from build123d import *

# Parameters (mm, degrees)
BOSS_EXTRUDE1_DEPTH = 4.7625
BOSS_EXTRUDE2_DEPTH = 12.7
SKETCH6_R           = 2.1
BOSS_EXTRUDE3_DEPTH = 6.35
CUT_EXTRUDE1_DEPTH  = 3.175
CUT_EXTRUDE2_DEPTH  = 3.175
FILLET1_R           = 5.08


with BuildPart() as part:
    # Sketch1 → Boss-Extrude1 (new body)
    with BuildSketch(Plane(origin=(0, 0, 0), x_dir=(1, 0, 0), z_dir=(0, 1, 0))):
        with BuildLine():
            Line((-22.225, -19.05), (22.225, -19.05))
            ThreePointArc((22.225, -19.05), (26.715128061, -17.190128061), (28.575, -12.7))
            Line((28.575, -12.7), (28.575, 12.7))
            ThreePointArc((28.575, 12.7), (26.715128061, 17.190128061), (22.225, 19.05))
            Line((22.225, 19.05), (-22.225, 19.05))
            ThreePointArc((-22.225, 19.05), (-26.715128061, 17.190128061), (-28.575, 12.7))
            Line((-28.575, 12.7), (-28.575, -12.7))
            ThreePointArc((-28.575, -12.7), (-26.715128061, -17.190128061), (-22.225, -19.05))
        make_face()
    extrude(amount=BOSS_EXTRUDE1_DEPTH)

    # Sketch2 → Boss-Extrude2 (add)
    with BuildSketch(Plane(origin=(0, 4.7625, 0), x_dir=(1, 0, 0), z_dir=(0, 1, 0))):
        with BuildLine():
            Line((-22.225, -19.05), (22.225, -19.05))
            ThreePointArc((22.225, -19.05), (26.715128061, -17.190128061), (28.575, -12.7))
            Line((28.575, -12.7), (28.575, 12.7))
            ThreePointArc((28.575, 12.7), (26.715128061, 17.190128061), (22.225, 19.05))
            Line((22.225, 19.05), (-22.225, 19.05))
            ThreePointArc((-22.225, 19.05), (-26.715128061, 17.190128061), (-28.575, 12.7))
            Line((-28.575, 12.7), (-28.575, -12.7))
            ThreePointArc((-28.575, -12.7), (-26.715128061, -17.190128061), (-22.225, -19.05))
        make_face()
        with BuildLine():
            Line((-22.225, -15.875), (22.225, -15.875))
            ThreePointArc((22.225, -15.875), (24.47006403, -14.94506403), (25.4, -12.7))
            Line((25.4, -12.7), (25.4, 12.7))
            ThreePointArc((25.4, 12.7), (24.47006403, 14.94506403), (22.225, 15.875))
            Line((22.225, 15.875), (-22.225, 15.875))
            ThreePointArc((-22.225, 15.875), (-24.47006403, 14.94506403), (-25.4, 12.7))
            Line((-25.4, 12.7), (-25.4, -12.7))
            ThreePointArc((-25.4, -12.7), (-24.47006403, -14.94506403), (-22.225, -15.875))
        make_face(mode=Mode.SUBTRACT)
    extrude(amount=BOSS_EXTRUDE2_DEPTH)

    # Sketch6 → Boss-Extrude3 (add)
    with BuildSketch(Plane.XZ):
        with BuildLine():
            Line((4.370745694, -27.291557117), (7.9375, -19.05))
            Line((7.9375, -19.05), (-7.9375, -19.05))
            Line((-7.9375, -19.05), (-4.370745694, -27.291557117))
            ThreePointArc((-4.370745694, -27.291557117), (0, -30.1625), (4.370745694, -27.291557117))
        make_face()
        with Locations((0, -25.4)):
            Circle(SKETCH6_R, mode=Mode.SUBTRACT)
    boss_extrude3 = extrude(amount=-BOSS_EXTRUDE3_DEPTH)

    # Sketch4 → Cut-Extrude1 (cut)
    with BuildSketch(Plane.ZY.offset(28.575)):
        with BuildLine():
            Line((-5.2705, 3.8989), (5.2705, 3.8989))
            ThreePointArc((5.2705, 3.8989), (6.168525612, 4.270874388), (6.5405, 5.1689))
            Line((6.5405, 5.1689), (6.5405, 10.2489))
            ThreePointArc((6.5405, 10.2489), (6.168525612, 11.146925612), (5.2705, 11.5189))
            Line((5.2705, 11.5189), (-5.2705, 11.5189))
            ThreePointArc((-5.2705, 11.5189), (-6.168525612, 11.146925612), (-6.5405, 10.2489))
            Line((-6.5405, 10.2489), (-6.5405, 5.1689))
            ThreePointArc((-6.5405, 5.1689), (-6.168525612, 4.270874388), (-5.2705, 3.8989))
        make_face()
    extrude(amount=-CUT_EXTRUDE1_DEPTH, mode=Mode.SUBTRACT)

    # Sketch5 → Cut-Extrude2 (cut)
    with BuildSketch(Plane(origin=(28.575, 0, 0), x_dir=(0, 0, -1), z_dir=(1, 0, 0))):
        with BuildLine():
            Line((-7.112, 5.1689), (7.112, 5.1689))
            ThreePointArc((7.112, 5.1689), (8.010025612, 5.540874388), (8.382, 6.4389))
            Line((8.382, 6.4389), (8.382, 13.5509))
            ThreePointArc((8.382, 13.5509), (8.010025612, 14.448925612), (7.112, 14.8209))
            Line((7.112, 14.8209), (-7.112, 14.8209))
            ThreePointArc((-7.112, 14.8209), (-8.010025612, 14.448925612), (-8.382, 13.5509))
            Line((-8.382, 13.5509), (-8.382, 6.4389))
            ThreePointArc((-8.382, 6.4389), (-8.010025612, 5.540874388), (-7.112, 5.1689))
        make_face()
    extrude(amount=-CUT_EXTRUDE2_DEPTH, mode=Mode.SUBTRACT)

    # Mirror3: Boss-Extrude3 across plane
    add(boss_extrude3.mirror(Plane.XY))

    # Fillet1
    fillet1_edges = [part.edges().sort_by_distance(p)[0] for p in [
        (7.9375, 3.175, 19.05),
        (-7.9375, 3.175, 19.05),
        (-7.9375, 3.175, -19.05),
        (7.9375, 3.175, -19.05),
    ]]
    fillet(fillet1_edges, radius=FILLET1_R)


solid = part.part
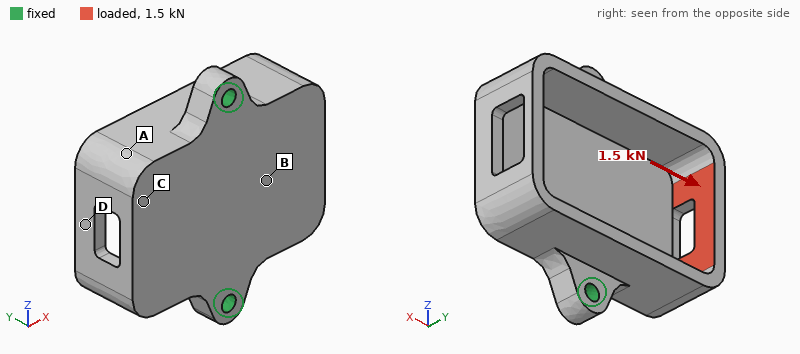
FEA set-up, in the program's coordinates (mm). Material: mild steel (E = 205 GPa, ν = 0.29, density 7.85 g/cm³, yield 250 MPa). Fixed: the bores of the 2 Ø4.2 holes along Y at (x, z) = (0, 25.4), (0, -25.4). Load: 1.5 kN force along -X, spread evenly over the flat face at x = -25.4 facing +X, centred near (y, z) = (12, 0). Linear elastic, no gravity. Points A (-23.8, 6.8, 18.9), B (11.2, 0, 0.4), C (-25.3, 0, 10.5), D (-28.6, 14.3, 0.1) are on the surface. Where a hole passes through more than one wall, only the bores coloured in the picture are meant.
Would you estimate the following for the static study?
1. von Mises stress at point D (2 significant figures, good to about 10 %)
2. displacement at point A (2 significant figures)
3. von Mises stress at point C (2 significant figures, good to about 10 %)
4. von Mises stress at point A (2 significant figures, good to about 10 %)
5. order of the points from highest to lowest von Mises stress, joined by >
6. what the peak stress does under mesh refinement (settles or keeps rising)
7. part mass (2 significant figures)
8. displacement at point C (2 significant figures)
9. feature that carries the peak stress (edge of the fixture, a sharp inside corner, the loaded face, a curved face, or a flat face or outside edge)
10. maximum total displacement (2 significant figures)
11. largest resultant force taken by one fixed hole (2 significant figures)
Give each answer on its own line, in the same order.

140 MPa
20 µm
29 MPa
43 MPa
D > A > C > B
keeps rising
140 g
23 µm
a sharp inside corner
62 µm
760 N
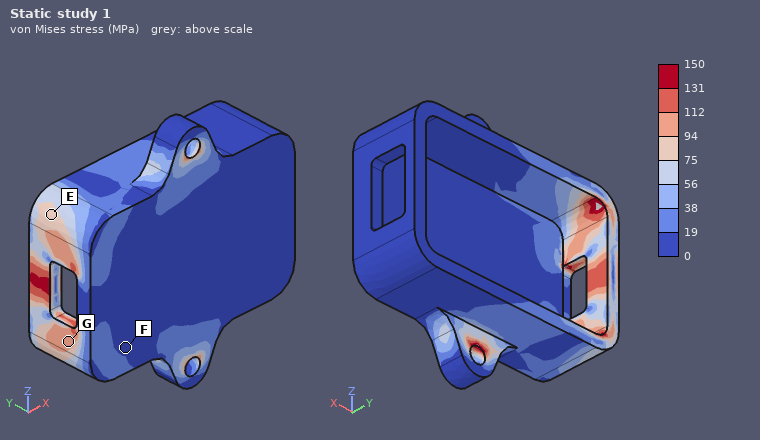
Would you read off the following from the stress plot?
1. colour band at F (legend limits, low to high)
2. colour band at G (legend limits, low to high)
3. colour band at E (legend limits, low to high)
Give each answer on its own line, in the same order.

0 to 19 MPa
94 to 112 MPa
75 to 94 MPa
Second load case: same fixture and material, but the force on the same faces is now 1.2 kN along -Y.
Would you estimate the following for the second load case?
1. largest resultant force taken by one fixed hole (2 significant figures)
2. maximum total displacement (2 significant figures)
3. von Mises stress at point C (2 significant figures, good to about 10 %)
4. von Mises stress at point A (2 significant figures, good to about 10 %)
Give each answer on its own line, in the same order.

610 N
64 µm
21 MPa
25 MPa
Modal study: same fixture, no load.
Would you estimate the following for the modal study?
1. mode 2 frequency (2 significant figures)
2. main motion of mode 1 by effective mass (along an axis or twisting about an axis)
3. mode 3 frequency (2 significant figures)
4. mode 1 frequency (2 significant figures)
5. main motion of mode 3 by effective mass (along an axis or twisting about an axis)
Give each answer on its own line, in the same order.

6600 Hz
twisting about Z
7100 Hz
3300 Hz
along Y
